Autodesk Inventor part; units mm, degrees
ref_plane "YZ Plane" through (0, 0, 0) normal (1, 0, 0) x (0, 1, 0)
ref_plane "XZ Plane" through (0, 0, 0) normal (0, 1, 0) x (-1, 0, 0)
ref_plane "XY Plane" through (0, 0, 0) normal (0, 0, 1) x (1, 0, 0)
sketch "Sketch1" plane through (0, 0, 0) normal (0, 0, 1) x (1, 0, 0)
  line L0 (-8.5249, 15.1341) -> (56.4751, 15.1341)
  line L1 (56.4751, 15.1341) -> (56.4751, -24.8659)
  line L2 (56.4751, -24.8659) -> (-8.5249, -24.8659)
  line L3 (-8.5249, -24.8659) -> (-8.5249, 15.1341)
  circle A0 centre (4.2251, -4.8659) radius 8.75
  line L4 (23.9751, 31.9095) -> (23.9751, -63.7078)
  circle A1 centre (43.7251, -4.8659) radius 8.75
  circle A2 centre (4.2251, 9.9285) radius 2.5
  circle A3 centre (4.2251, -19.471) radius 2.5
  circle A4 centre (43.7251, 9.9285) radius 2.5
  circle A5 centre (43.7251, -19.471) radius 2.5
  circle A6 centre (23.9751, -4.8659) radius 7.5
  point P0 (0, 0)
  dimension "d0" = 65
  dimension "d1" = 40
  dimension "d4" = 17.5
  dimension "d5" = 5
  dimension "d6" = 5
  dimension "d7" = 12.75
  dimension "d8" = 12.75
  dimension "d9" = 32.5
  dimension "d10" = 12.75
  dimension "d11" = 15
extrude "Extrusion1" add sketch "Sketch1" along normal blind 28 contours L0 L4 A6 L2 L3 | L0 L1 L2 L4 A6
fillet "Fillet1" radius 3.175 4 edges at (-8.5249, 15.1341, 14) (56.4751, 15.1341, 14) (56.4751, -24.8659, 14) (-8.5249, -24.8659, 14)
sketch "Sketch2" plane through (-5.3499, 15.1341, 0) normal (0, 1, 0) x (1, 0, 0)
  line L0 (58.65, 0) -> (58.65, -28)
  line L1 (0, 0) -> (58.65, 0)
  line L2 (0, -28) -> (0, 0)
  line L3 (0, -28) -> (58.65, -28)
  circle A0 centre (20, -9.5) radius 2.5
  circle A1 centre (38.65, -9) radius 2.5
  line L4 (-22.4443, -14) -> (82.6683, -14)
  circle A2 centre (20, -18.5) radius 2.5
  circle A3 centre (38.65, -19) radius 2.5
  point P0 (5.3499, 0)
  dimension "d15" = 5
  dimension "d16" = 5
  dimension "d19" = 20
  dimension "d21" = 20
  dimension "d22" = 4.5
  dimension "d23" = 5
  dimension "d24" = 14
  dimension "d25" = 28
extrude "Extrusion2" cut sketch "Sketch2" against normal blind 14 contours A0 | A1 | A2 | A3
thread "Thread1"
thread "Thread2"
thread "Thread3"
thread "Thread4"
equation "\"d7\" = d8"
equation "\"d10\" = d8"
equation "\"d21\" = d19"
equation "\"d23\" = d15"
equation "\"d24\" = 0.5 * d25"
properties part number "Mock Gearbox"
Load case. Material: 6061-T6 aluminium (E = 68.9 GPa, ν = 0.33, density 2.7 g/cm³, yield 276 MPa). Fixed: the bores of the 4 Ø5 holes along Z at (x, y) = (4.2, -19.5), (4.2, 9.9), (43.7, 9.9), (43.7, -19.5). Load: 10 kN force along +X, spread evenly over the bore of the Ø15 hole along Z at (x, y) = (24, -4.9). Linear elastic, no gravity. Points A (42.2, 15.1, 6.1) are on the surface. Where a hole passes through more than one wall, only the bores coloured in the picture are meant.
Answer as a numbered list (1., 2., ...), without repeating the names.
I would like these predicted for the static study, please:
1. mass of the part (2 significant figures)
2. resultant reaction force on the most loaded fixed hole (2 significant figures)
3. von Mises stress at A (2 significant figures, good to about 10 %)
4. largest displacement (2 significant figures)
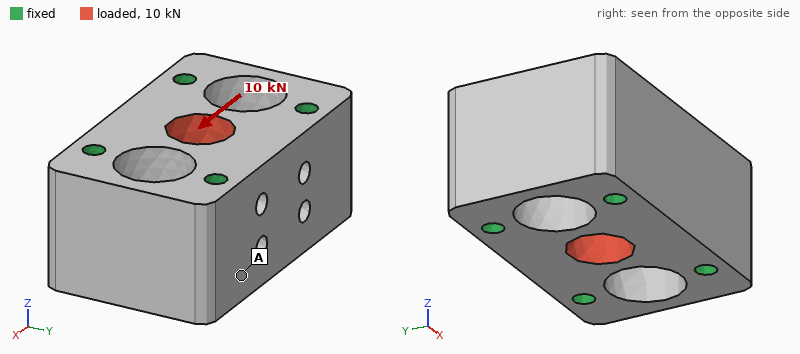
1. 140 g
2. 2.8 kN
3. 3.3 MPa
4. 4.3 µm
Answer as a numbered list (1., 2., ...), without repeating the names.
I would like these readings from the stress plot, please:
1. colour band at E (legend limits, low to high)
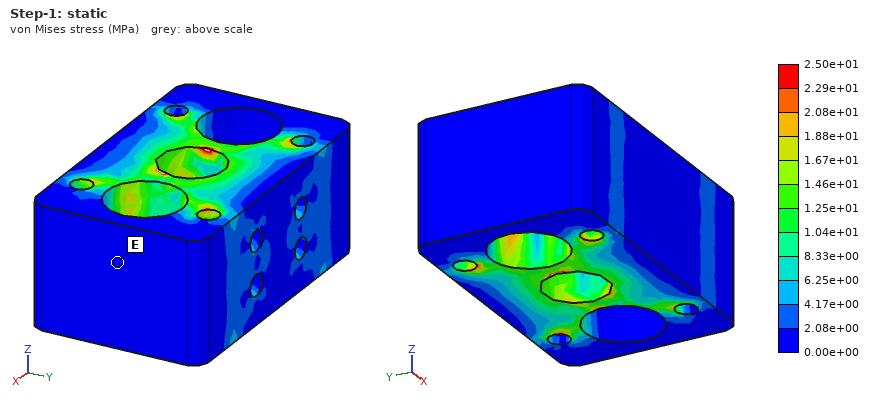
1. 0.00e+00 to 2.08e+00 MPa
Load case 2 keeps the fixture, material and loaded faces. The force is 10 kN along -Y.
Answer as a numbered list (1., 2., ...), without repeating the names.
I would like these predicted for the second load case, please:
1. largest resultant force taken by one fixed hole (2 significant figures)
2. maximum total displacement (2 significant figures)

1. 2.9 kN
2. 6.8 µm
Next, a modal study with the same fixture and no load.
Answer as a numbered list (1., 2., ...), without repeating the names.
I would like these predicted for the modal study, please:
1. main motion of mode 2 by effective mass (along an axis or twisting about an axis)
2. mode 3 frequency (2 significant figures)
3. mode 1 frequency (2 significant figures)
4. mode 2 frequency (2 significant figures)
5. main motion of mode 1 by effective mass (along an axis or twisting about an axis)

1. along Z
2. 34 kHz
3. 28 kHz
4. 31 kHz
5. along Y
